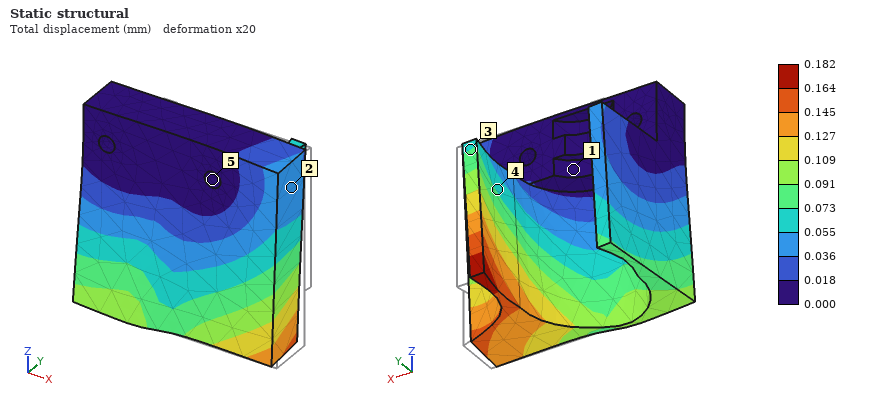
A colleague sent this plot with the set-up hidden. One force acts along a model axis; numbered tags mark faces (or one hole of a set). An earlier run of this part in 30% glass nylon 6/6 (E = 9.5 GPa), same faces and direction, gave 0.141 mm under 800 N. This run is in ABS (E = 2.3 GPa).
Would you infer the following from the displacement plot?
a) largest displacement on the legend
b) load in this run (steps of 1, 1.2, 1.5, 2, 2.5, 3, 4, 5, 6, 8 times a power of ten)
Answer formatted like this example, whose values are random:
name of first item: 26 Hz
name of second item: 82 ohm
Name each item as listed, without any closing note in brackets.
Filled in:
largest displacement on the legend: 0.182 mm
load in this run: 250 N
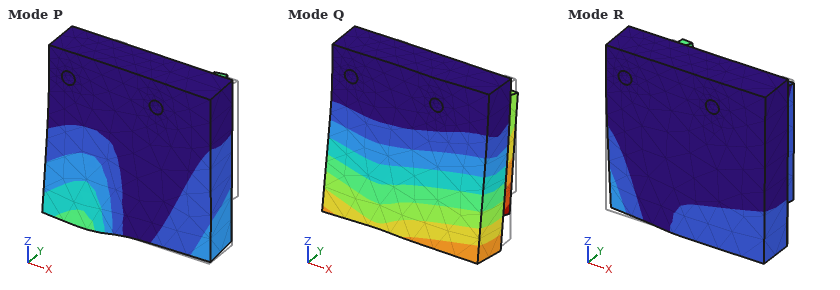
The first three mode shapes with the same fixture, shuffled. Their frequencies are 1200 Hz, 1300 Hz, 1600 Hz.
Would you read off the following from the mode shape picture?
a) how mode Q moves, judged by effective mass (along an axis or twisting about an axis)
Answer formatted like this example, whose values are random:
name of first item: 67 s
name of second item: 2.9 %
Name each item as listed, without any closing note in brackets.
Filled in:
how mode Q moves, judged by effective mass: along Y
